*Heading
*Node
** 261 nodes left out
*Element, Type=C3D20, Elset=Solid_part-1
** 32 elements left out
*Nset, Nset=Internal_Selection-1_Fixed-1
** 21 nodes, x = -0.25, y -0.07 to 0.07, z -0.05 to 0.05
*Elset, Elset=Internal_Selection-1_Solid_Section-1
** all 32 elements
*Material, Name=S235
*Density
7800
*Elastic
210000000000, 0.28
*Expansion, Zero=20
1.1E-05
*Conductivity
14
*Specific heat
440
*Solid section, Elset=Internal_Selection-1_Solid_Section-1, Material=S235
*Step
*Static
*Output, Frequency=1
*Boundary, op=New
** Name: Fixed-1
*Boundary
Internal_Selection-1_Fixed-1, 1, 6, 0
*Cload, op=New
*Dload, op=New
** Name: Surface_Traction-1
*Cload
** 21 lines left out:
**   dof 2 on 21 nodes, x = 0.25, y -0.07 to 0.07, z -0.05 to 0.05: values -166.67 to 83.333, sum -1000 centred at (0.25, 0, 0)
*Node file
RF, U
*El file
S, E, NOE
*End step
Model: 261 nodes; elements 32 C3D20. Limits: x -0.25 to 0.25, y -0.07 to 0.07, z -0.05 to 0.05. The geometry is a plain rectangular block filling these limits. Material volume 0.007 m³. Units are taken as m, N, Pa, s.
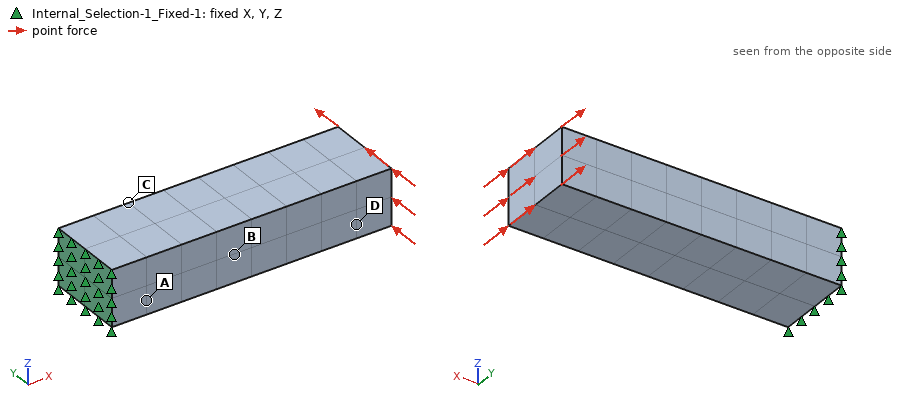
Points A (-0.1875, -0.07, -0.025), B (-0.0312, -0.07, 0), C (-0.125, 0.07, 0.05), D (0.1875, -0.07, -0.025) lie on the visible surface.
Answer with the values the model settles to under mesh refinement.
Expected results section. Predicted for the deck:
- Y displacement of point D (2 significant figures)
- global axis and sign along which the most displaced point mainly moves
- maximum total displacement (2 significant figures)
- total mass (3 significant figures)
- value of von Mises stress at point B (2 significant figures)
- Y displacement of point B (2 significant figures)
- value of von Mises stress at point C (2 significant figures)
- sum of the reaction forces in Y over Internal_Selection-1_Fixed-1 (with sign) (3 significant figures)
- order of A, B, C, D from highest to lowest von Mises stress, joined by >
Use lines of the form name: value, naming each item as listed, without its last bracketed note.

Y displacement of point D: -7.4e-06 m
global axis and sign along which the most displaced point mainly moves: -Y
maximum total displacement: 9.4e-06 m
total mass: 54.6 kg
value of von Mises stress at point B: 8.6e+05 Pa
Y displacement of point B: -2.3e-06 m
value of von Mises stress at point C: 1.1e+06 Pa
sum of the reaction forces in Y over Internal_Selection-1_Fixed-1 (with sign): 1000 N
order of A, B, C, D from highest to lowest von Mises stress, joined by >: A > C > B > D
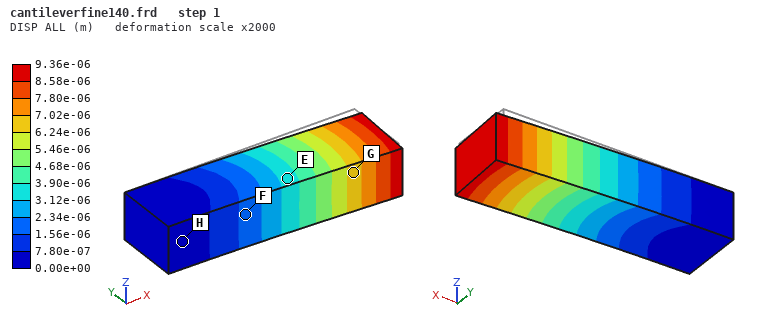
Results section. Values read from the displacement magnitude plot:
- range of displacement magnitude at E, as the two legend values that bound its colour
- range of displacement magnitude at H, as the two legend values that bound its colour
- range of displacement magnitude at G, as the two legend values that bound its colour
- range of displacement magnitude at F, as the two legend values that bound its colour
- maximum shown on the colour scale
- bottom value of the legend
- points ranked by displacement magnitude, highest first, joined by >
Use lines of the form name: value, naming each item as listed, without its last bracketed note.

range of displacement magnitude at E, as the two legend values that bound its colour: 3.12e-06 to 3.90e-06 m
range of displacement magnitude at H, as the two legend values that bound its colour: 0.00e+00 to 7.80e-07 m
range of displacement magnitude at G, as the two legend values that bound its colour: 6.24e-06 to 7.02e-06 m
range of displacement magnitude at F, as the two legend values that bound its colour: 1.56e-06 to 2.34e-06 m
maximum shown on the colour scale: 9.36e-06 m
bottom value of the legend: 0.00e+00 m
points ranked by displacement magnitude, highest first, joined by >: G > E > F > H
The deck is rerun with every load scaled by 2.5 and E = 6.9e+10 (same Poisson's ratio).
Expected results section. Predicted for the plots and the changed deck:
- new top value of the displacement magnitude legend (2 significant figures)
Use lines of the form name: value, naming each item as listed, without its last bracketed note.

new top value of the displacement magnitude legend: 7.1e-05 m
